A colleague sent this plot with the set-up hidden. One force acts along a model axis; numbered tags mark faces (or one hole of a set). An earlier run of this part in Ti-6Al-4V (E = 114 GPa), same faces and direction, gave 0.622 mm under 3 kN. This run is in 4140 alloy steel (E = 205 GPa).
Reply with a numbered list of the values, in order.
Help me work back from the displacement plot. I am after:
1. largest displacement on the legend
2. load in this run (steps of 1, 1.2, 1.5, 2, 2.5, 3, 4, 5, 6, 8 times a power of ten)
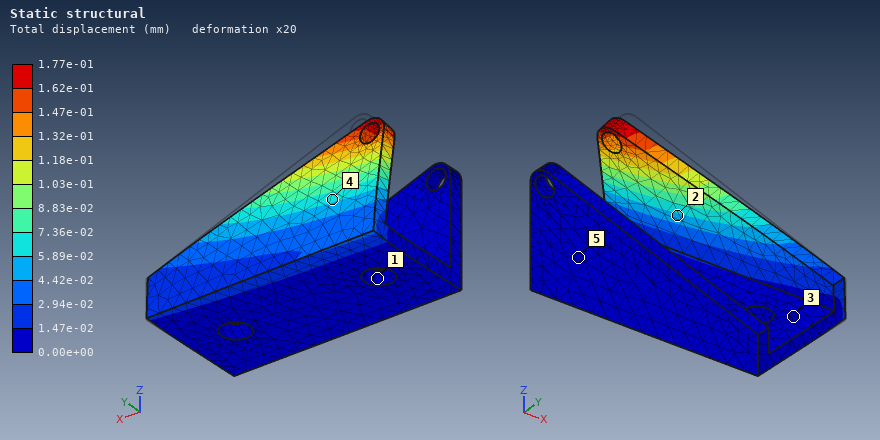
1. 1.77e-01 mm
2. 1.5 kN
